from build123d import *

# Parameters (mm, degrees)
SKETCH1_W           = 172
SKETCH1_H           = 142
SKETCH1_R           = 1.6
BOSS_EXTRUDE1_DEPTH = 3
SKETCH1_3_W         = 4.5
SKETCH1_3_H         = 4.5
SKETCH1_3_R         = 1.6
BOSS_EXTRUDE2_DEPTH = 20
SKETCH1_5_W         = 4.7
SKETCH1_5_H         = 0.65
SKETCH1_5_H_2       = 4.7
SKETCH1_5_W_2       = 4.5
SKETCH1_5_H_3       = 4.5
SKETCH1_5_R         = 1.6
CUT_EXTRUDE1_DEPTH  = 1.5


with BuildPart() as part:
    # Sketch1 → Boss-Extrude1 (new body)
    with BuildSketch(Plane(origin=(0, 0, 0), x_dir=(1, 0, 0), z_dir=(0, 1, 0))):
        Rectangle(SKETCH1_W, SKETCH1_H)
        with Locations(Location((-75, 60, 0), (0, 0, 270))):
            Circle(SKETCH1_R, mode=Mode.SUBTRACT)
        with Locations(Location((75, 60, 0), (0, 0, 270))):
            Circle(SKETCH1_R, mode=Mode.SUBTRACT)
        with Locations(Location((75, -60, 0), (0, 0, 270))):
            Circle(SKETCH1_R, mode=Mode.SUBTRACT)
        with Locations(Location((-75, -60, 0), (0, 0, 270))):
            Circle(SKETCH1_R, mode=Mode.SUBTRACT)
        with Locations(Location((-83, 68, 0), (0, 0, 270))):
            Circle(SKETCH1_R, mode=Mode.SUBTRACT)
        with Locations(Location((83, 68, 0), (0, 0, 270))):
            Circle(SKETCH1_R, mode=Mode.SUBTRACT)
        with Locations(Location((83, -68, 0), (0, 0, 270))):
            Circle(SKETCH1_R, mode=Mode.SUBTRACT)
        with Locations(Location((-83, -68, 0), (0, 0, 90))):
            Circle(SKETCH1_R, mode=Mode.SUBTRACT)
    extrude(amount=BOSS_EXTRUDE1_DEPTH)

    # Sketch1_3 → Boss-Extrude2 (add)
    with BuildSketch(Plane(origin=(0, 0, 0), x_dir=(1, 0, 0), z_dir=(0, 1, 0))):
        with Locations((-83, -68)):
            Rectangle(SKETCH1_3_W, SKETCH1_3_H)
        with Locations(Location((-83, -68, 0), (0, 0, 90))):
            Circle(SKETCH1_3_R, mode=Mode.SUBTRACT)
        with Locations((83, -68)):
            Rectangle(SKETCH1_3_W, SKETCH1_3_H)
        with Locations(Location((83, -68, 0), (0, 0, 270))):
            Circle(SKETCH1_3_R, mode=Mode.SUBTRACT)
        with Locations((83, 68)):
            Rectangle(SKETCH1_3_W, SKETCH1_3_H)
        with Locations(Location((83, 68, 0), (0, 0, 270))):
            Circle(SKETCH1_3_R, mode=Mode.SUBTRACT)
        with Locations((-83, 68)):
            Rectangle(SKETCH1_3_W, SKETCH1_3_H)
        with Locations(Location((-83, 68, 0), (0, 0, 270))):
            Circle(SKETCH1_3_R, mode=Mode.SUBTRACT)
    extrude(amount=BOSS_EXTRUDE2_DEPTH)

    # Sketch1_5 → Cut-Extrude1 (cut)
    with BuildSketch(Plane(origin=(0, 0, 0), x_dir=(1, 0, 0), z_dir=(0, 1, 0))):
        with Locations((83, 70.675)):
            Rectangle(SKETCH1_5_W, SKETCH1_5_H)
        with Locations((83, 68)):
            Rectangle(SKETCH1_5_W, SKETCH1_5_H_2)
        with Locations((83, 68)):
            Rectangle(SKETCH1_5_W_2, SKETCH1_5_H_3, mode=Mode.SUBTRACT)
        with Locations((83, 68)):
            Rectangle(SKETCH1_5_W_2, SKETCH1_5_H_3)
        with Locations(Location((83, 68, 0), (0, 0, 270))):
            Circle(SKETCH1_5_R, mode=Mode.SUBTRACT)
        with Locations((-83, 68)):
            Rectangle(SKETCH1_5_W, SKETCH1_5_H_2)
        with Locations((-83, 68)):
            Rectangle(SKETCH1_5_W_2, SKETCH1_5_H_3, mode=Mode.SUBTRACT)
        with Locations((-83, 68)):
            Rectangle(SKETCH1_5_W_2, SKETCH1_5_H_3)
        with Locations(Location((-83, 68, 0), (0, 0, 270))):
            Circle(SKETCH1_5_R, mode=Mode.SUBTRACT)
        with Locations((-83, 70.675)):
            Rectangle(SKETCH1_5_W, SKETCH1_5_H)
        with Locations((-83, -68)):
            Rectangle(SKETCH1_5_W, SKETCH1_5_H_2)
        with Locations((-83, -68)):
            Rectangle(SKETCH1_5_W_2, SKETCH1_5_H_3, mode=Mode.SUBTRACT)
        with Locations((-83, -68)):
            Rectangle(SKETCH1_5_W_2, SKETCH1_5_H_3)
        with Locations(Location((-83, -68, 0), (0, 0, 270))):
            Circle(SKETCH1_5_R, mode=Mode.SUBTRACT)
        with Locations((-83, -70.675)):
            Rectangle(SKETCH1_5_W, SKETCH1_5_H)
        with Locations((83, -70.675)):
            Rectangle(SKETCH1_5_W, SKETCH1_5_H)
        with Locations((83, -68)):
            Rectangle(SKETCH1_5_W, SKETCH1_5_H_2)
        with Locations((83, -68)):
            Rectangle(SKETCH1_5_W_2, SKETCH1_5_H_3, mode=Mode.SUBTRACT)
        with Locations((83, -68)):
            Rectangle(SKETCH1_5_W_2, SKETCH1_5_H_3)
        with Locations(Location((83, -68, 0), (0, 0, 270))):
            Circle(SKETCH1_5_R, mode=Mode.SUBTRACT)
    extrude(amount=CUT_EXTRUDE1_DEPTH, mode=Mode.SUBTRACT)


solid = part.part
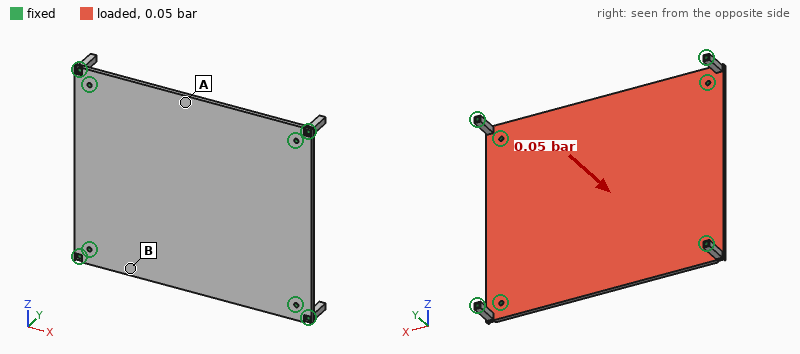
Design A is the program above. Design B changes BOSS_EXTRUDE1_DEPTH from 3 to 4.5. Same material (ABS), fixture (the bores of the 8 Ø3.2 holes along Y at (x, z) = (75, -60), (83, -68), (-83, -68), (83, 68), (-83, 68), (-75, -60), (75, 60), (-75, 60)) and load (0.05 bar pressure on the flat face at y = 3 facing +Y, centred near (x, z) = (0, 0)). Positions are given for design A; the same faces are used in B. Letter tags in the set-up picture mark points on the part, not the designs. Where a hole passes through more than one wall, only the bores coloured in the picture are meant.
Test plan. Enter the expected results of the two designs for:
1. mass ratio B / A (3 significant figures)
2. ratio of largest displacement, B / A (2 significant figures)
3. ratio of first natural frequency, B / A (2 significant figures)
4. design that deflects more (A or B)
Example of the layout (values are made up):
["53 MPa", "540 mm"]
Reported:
["1.49", "0.31", "1.5", "A"]
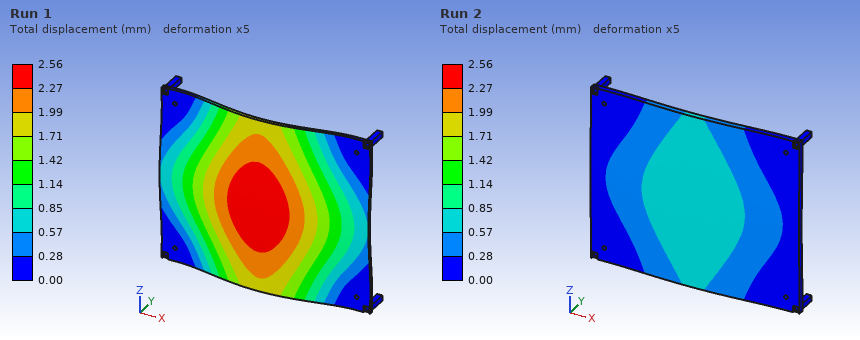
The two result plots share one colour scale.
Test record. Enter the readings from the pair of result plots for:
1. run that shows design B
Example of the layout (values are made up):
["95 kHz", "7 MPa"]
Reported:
["Run 2"]
